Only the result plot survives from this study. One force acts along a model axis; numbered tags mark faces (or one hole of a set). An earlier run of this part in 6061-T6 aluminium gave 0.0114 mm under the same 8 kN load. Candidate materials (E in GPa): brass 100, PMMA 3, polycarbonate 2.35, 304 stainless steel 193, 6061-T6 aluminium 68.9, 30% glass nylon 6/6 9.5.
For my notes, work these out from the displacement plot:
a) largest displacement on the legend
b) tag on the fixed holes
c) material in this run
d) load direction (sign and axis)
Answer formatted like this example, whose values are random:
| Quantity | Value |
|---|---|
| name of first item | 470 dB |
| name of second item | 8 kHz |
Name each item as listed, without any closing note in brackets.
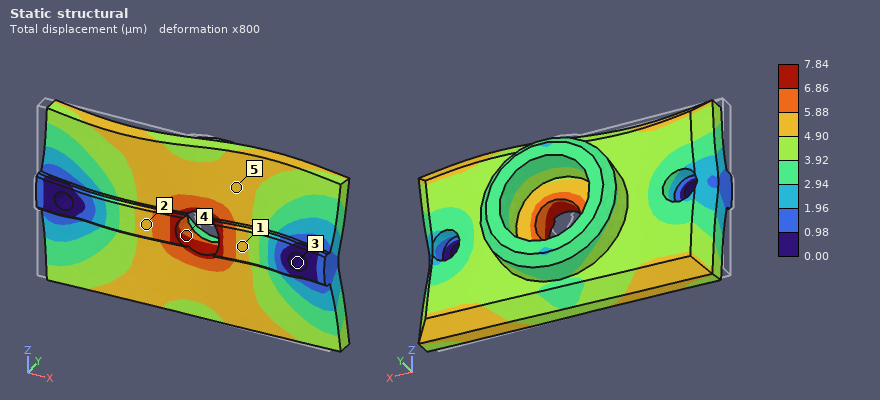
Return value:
| Quantity | Value |
|---|---|
| largest displacement on the legend | 7.84 µm |
| tag on the fixed holes | 3 |
| material in this run | brass |
| load direction | +X |
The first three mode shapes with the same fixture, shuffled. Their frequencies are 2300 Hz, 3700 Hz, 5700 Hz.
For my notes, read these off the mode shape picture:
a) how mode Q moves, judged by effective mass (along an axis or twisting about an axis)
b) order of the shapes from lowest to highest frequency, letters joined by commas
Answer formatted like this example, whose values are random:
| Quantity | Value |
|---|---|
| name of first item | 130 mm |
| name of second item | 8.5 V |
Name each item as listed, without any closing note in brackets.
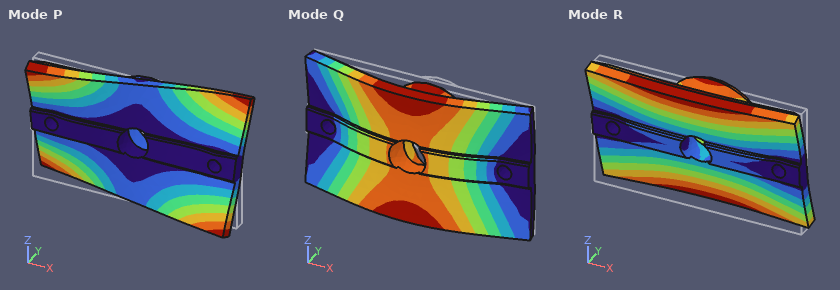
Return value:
| Quantity | Value |
|---|---|
| how mode Q moves, judged by effective mass | along Y |
| order of the shapes from lowest to highest frequency, letters joined by commas | R, Q, P |
